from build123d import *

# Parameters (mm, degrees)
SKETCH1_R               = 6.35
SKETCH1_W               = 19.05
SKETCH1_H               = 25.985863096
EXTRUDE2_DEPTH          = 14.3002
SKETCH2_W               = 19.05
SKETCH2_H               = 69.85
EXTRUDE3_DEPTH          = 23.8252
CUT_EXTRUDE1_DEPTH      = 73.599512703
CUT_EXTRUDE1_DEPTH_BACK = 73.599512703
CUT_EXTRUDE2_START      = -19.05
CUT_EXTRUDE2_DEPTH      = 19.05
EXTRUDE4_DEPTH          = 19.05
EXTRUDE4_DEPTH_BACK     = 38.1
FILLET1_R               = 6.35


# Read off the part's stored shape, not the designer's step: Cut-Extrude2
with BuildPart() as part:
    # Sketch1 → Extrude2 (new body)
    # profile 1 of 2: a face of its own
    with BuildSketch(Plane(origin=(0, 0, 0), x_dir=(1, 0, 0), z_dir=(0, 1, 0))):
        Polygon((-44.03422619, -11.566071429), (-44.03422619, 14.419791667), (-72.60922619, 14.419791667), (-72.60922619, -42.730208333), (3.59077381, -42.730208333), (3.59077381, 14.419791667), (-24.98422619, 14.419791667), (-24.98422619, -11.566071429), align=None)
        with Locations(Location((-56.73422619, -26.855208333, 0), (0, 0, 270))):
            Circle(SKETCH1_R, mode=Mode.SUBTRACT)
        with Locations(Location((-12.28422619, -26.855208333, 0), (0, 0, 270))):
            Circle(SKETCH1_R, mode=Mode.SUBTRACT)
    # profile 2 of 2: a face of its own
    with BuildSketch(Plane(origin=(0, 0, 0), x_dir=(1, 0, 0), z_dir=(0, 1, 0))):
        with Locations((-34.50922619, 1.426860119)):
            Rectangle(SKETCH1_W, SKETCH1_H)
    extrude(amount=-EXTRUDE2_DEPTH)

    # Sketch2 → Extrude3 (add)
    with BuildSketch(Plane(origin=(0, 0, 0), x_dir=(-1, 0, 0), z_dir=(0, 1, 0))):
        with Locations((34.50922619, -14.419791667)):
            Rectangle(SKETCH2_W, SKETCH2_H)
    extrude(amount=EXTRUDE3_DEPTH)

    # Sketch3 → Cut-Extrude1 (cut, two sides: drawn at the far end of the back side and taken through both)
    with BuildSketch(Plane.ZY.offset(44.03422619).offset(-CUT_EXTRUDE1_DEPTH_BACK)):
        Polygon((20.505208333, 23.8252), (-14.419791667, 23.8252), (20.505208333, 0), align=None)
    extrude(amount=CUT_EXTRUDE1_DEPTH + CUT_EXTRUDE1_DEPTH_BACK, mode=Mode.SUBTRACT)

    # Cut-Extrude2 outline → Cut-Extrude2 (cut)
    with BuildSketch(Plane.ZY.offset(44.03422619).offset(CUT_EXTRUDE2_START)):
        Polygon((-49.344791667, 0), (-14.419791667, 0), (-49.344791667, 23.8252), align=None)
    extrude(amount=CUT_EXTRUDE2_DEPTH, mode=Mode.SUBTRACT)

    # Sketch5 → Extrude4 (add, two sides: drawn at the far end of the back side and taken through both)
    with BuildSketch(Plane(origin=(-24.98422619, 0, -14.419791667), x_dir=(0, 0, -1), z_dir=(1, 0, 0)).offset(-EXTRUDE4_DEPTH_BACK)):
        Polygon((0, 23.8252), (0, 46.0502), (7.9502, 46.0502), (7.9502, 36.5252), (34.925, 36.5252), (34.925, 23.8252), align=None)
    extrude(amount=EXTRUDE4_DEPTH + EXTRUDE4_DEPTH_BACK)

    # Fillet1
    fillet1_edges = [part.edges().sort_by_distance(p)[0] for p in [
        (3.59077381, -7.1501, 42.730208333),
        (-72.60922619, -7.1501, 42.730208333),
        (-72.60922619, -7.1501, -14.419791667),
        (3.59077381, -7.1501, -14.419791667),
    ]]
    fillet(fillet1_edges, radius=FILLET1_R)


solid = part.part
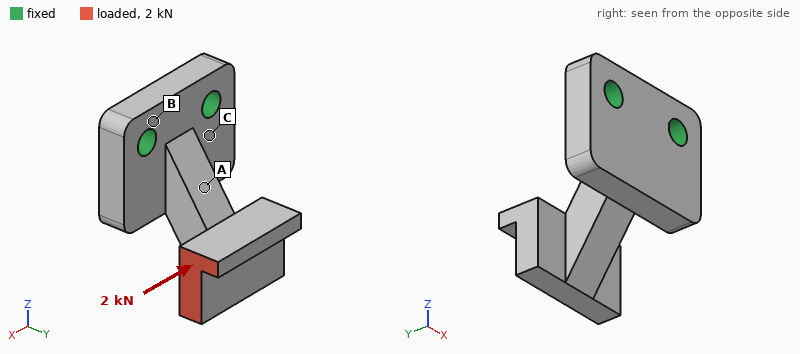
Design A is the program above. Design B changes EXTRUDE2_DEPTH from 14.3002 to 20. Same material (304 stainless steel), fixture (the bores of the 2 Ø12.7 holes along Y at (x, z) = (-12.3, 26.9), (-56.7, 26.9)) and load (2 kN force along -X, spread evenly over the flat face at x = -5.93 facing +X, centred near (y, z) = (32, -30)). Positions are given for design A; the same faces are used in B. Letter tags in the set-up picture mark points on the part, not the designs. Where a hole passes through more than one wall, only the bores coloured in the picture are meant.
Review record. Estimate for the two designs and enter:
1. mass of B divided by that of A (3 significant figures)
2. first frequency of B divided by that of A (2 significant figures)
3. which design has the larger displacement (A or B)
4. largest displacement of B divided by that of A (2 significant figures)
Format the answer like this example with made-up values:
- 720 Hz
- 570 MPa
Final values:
- 1.22
- 1.3
- A
- 0.89
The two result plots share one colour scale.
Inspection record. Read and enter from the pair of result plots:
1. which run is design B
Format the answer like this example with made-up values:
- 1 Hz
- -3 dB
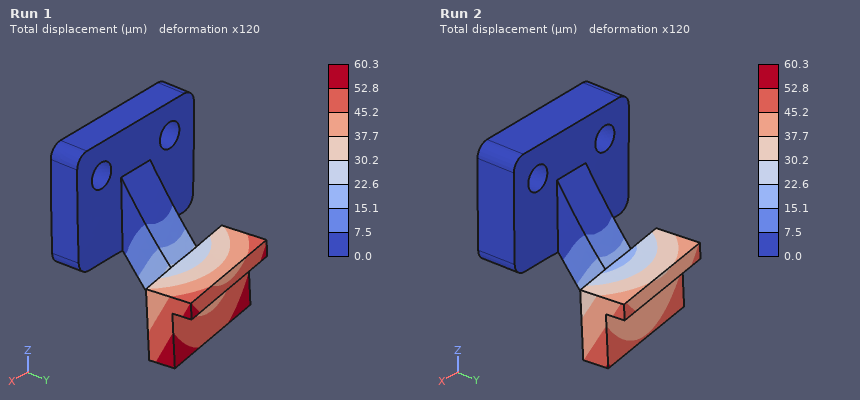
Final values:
- Run 2
